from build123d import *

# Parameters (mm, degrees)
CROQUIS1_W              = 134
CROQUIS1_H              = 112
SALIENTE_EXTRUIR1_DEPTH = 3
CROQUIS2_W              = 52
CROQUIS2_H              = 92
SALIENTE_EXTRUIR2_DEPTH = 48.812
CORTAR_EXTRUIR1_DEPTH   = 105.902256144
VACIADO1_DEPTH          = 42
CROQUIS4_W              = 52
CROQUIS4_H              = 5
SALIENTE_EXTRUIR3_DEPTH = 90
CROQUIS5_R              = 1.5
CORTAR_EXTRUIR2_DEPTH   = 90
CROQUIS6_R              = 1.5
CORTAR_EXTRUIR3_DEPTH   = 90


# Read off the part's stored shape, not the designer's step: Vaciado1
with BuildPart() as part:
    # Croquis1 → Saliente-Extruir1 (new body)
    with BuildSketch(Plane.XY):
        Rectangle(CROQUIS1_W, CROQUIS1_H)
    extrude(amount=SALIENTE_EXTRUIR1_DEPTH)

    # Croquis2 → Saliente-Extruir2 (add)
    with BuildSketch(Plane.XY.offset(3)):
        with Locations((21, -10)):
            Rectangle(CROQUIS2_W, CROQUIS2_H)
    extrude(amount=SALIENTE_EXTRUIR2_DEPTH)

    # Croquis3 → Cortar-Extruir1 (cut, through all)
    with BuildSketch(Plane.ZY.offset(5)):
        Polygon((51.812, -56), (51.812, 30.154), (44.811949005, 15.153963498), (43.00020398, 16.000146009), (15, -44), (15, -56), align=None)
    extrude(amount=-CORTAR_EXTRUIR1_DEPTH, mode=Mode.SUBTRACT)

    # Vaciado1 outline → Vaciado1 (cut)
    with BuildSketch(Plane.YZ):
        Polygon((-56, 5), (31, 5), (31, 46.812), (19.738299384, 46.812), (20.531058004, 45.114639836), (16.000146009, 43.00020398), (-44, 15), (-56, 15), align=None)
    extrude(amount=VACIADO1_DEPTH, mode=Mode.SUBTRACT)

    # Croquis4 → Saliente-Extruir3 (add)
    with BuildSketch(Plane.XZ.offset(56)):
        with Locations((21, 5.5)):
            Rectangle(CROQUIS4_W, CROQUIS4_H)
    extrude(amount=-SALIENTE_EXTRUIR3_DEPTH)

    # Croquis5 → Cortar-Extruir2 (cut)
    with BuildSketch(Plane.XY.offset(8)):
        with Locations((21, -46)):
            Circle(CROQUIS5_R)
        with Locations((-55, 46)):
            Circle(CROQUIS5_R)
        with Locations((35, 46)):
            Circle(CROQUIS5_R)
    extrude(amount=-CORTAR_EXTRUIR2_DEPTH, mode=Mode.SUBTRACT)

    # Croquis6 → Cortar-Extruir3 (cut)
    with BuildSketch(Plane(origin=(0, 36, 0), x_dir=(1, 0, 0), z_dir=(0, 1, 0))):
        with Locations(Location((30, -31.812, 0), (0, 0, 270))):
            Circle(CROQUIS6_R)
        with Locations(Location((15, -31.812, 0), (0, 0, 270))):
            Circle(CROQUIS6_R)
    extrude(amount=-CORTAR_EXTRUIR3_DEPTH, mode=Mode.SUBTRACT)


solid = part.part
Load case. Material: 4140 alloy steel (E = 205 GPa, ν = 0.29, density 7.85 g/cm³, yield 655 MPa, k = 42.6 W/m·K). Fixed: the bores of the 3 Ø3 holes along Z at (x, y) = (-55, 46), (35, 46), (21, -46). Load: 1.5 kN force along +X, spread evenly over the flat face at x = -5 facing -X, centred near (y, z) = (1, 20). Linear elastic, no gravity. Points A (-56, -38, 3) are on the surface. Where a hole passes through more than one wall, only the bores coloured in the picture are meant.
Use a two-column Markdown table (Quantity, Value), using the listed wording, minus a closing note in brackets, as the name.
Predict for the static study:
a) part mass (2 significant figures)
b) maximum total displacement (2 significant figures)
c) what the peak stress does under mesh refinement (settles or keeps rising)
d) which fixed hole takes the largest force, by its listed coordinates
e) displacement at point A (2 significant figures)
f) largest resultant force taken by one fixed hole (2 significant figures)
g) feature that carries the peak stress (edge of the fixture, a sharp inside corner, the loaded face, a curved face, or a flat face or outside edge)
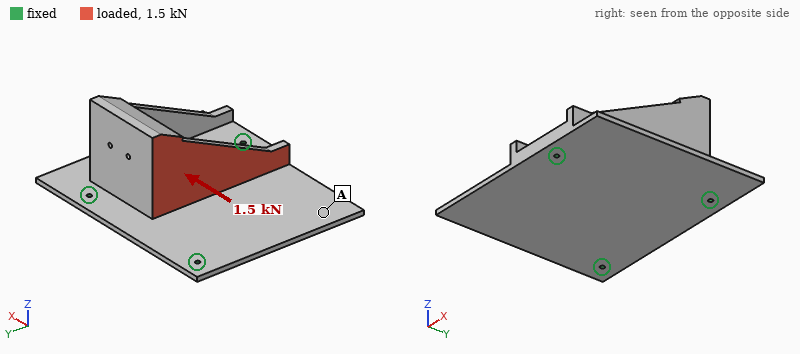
| Quantity | Value |
|---|---|
| part mass | 800 g |
| maximum total displacement | 71 µm |
| what the peak stress does under mesh refinement | keeps rising |
| which fixed hole takes the largest force, by its listed coordinates | (21, -46) |
| displacement at point A | 37 µm |
| largest resultant force taken by one fixed hole | 1.1 kN |
| feature that carries the peak stress | edge of the fixture |
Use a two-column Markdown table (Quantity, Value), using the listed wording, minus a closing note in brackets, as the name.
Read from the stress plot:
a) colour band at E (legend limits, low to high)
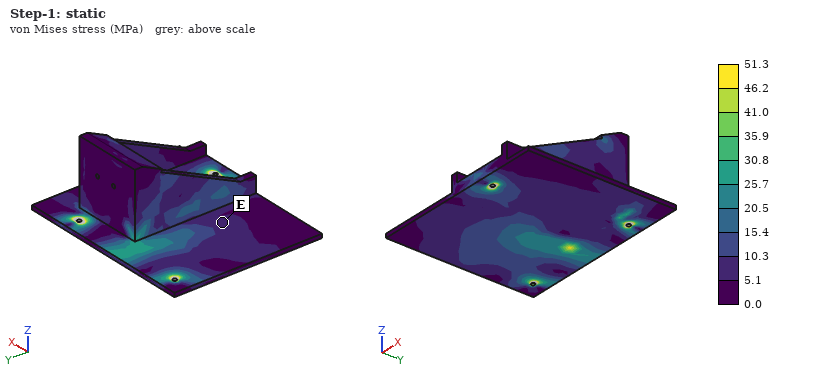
| Quantity | Value |
|---|---|
| colour band at E | 5.1 to 10.3 MPa |
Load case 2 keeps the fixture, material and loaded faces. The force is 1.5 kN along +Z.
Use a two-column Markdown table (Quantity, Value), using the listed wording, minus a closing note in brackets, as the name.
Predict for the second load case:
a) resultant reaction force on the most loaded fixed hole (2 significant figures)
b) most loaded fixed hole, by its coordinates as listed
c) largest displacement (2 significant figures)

| Quantity | Value |
|---|---|
| resultant reaction force on the most loaded fixed hole | 1.1 kN |
| most loaded fixed hole, by its coordinates as listed | (21, -46) |
| largest displacement | 0.12 mm |
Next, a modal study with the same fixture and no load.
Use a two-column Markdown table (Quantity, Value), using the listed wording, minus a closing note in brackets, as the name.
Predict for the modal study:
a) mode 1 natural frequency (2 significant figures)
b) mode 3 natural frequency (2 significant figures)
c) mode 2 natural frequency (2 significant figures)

| Quantity | Value |
|---|---|
| mode 1 natural frequency | 780 Hz |
| mode 3 natural frequency | 2100 Hz |
| mode 2 natural frequency | 1200 Hz |
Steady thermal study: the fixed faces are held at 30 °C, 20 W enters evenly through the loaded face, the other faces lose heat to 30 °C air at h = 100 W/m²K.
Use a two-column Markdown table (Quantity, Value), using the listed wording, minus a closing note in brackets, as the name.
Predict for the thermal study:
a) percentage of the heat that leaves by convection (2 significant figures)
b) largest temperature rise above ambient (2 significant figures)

| Quantity | Value |
|---|---|
| percentage of the heat that leaves by convection | 83 % |
| largest temperature rise above ambient | 17 K |
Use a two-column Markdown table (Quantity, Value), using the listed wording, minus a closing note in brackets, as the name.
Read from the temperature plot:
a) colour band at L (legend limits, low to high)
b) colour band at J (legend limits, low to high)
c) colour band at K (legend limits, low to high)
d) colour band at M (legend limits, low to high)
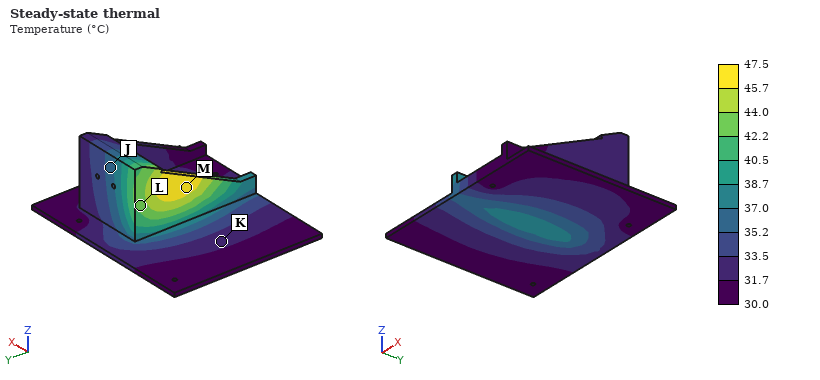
| Quantity | Value |
|---|---|
| colour band at L | 42.2 to 44.0 °C |
| colour band at J | 35.2 to 37.0 °C |
| colour band at K | 31.7 to 33.5 °C |
| colour band at M | 45.7 to 47.5 °C |
